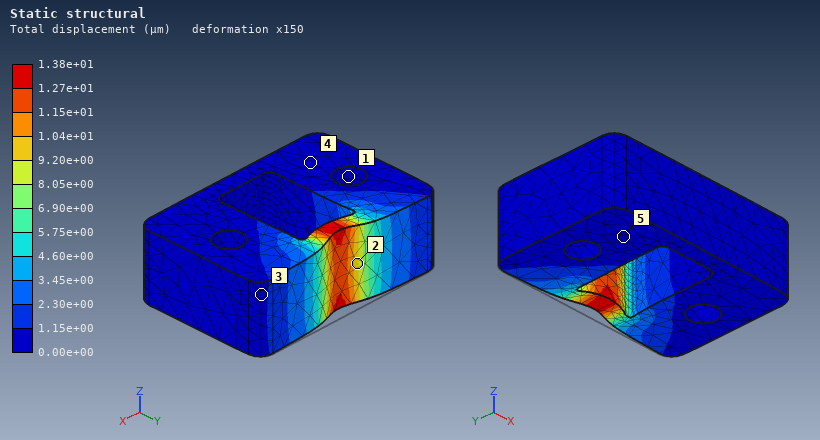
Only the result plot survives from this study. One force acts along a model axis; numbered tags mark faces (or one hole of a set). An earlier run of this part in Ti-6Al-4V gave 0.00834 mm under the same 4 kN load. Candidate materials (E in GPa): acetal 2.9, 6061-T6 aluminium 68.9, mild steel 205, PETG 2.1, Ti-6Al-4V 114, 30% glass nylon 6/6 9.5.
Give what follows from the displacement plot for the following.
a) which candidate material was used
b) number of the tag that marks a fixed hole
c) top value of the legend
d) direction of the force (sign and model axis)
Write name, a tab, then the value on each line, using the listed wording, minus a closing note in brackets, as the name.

which candidate material was used	6061-T6 aluminium
number of the tag that marks a fixed hole	1
top value of the legend	1.38e+01 µm
direction of the force	-Y
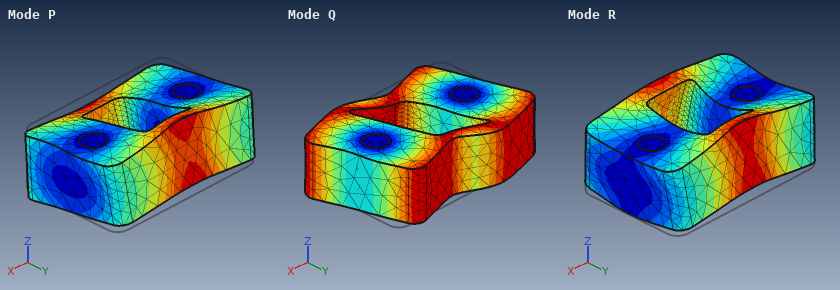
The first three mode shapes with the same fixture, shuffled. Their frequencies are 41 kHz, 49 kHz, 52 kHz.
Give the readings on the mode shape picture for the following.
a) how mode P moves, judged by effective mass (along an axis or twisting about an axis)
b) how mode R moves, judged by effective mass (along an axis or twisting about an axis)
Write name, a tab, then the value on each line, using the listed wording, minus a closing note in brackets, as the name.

how mode P moves, judged by effective mass	twisting about X
how mode R moves, judged by effective mass	along Z
